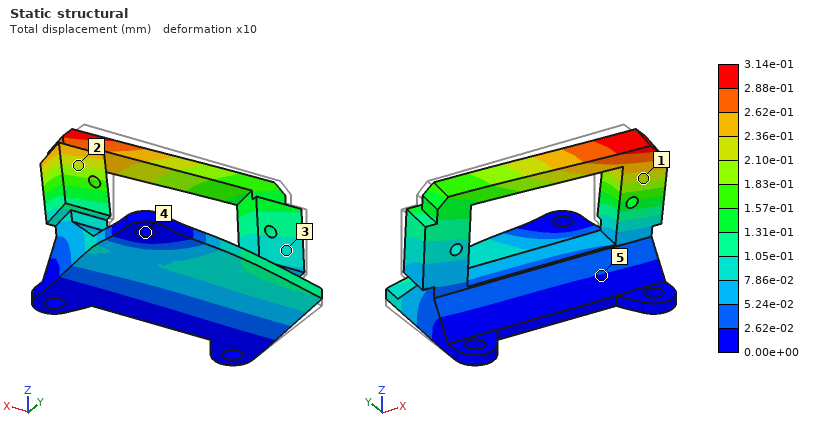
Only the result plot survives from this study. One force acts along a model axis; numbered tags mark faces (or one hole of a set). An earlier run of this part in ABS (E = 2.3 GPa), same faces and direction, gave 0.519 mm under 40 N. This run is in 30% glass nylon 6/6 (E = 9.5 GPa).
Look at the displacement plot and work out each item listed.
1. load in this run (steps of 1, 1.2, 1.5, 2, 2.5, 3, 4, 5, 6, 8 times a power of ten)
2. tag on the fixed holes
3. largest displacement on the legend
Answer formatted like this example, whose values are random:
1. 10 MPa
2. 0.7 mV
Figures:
1. 100 N
2. 4
3. 3.14e-01 mm
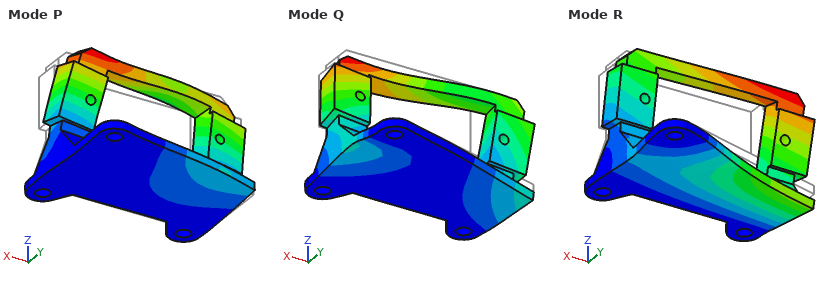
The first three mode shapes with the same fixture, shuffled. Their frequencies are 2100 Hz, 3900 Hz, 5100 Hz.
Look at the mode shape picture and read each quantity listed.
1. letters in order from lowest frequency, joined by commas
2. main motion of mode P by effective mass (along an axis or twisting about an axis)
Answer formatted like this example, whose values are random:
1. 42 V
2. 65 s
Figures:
1. R, Q, P
2. along X
